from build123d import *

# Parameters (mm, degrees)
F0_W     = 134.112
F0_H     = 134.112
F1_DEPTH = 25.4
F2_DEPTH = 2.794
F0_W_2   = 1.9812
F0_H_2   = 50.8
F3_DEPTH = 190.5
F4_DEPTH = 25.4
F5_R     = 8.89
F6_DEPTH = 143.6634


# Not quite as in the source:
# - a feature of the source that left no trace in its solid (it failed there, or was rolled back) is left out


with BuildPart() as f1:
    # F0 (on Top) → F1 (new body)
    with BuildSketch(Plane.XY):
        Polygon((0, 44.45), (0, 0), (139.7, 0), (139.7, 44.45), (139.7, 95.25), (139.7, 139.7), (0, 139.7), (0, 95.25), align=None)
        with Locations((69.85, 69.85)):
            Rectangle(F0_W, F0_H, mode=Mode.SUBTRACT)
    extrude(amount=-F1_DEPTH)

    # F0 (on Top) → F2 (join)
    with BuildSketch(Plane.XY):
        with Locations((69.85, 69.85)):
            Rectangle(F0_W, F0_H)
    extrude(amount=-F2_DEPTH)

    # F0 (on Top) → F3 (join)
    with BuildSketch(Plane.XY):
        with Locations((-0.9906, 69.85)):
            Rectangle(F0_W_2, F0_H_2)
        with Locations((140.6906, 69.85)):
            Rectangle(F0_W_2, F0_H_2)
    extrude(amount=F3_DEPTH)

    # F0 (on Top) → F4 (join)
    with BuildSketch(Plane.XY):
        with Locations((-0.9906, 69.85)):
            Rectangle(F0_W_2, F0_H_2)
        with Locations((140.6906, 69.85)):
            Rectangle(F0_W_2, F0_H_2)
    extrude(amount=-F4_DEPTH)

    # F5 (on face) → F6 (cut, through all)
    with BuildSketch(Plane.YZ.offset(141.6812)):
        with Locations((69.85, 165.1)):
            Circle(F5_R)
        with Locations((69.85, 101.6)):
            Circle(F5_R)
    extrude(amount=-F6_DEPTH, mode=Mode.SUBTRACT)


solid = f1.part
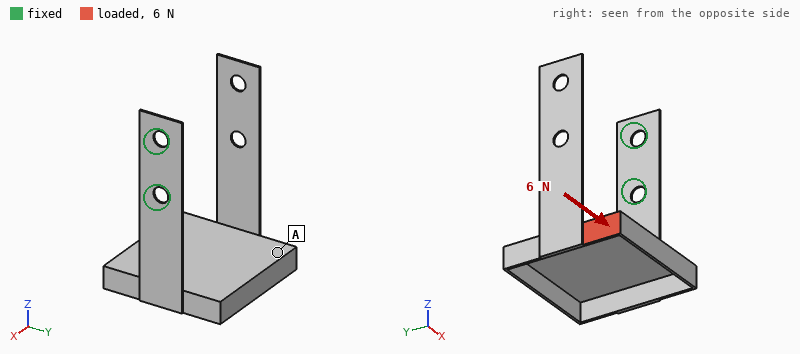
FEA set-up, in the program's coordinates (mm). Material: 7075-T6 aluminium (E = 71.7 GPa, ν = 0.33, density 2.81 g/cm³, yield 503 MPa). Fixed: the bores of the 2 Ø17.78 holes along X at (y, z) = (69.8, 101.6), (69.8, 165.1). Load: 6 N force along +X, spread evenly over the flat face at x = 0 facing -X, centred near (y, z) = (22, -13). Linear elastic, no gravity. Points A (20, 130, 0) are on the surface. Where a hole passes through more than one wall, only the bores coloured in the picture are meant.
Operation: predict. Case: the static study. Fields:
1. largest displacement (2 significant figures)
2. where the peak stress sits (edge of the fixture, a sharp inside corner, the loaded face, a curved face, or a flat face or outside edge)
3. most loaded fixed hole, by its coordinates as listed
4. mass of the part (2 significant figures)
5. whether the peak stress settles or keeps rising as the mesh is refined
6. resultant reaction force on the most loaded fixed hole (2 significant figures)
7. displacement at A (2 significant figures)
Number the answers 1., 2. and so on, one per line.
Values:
1. 3.0 mm
2. edge of the fixture
3. (69.8, 101.6)
4. 370 g
5. keeps rising
6. 5.9 N
7. 1.9 mm
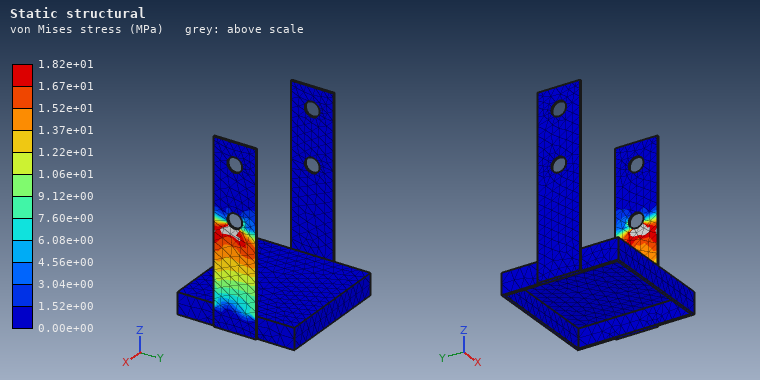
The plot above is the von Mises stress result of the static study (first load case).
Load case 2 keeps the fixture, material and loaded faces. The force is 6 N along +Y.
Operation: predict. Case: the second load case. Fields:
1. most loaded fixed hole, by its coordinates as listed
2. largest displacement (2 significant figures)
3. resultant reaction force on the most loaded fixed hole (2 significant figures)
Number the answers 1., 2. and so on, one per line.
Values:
1. (69.8, 101.6)
2. 3.0 mm
3. 11 N
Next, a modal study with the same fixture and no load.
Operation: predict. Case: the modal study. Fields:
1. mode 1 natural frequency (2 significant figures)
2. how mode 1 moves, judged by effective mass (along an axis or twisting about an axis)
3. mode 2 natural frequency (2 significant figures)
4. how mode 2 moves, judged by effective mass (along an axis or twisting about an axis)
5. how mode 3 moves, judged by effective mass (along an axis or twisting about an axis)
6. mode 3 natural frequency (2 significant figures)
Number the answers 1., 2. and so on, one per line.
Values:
1. 12 Hz
2. along Z
3. 18 Hz
4. along Y
5. along X
6. 41 Hz
